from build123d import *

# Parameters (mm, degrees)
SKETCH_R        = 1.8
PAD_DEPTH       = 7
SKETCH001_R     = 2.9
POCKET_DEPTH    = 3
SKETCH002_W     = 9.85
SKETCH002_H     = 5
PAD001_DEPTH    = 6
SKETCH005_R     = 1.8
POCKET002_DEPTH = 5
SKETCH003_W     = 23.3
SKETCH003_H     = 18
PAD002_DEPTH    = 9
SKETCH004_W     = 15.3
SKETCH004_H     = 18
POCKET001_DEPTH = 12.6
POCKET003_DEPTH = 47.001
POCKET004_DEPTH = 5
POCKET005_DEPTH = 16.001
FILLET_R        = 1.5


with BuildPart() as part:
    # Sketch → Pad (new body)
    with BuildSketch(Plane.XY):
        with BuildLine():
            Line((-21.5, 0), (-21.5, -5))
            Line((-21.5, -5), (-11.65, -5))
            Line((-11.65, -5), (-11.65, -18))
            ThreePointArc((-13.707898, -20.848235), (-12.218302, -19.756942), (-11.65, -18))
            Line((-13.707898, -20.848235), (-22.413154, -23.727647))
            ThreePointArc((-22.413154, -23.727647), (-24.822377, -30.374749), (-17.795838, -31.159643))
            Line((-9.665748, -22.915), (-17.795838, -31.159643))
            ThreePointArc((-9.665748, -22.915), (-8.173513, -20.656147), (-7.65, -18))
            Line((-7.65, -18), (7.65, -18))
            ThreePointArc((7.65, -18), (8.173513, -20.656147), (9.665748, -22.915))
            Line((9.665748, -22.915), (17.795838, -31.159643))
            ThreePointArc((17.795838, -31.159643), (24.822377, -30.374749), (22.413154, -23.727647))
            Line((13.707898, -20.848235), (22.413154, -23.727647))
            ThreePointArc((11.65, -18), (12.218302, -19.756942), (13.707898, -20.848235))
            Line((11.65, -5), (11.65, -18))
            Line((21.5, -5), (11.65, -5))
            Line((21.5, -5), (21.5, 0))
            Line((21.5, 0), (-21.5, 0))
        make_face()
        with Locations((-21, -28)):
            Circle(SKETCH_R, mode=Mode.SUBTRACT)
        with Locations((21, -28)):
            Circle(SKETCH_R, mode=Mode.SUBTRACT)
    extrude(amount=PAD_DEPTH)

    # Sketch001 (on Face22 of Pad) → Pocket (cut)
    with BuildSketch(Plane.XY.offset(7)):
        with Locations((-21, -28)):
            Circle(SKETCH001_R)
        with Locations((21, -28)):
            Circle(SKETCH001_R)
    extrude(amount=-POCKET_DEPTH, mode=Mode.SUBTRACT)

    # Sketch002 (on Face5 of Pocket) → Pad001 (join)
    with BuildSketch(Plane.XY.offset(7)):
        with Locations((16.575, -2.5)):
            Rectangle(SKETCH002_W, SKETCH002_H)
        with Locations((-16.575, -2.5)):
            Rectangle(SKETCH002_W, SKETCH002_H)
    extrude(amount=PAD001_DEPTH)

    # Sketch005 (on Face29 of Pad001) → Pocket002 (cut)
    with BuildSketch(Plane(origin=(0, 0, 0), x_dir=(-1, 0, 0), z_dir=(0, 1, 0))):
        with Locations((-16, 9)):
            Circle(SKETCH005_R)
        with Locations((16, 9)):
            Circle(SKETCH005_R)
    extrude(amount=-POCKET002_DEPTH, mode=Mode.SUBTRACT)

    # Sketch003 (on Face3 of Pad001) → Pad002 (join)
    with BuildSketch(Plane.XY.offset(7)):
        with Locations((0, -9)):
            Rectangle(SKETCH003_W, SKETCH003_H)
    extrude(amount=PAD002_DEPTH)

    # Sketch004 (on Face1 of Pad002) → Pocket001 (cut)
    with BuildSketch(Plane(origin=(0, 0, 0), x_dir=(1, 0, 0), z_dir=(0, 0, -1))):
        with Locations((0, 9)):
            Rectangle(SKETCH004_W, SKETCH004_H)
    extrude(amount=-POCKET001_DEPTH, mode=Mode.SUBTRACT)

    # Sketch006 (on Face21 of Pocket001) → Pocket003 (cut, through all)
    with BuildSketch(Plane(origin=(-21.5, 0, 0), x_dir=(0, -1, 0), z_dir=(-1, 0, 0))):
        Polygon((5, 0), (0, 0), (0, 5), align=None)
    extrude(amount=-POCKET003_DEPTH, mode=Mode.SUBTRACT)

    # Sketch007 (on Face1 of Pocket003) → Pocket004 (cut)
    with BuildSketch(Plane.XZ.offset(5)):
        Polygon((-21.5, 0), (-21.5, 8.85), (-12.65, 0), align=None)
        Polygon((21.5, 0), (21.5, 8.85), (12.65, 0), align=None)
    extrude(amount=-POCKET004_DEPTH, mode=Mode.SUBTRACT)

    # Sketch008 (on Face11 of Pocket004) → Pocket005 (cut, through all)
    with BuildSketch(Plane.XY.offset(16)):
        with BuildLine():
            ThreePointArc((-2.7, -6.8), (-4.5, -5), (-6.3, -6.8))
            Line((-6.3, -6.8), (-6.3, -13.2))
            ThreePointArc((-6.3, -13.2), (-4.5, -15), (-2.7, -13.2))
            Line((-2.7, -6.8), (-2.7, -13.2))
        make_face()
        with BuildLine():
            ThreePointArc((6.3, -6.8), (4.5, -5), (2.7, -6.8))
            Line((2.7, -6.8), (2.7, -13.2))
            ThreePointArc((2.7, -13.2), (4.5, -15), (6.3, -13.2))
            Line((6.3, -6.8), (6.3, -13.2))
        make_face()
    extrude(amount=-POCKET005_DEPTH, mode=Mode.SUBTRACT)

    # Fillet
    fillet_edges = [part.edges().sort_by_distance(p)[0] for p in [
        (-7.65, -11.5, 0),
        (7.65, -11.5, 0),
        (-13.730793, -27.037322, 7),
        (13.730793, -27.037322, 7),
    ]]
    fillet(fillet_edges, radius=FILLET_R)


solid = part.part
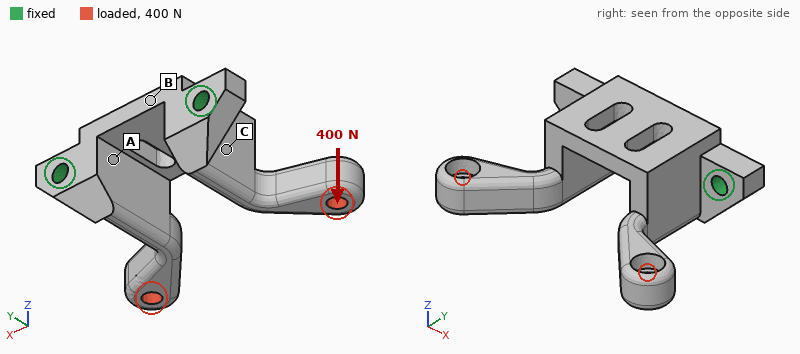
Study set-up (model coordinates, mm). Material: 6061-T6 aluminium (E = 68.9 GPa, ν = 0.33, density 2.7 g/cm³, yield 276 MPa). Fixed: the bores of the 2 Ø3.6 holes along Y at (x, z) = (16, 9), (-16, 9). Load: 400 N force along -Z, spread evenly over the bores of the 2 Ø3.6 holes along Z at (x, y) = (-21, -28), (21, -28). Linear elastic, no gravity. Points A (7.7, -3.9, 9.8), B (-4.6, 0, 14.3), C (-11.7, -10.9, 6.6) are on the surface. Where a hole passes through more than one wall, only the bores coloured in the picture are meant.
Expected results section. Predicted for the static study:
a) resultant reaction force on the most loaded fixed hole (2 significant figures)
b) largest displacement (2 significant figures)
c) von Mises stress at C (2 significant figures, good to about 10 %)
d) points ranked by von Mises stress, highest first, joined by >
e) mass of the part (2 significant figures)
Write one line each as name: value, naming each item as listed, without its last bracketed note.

resultant reaction force on the most loaded fixed hole: 260 N
largest displacement: 0.29 mm
von Mises stress at C: 59 MPa
points ranked by von Mises stress, highest first, joined by >: C > A > B
mass of the part: 14 g
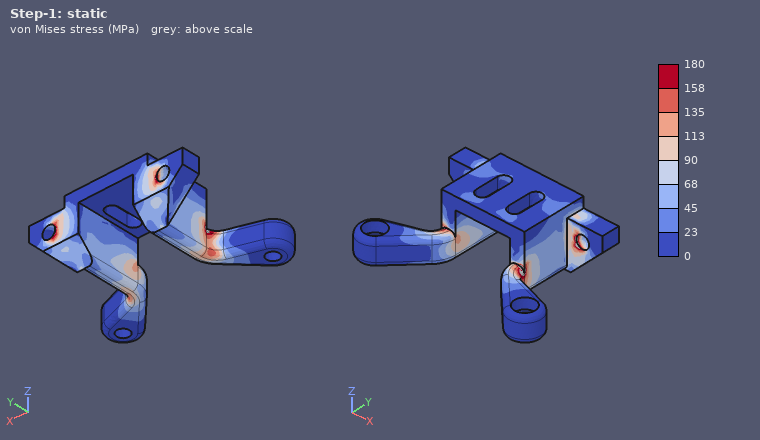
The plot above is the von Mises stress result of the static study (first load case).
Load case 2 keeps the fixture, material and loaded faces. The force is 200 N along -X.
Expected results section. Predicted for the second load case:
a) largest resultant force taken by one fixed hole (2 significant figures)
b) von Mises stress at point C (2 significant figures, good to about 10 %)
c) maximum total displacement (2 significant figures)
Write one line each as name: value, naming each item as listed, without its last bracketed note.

largest resultant force taken by one fixed hole: 180 N
von Mises stress at point C: 42 MPa
maximum total displacement: 0.18 mm
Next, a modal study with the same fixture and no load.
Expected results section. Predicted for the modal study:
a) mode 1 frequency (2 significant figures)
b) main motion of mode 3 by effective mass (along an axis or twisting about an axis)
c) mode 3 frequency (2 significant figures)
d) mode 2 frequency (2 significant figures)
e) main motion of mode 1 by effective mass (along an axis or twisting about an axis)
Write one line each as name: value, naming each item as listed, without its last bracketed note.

mode 1 frequency: 3300 Hz
main motion of mode 3 by effective mass: along Z
mode 3 frequency: 4200 Hz
mode 2 frequency: 3600 Hz
main motion of mode 1 by effective mass: along X
